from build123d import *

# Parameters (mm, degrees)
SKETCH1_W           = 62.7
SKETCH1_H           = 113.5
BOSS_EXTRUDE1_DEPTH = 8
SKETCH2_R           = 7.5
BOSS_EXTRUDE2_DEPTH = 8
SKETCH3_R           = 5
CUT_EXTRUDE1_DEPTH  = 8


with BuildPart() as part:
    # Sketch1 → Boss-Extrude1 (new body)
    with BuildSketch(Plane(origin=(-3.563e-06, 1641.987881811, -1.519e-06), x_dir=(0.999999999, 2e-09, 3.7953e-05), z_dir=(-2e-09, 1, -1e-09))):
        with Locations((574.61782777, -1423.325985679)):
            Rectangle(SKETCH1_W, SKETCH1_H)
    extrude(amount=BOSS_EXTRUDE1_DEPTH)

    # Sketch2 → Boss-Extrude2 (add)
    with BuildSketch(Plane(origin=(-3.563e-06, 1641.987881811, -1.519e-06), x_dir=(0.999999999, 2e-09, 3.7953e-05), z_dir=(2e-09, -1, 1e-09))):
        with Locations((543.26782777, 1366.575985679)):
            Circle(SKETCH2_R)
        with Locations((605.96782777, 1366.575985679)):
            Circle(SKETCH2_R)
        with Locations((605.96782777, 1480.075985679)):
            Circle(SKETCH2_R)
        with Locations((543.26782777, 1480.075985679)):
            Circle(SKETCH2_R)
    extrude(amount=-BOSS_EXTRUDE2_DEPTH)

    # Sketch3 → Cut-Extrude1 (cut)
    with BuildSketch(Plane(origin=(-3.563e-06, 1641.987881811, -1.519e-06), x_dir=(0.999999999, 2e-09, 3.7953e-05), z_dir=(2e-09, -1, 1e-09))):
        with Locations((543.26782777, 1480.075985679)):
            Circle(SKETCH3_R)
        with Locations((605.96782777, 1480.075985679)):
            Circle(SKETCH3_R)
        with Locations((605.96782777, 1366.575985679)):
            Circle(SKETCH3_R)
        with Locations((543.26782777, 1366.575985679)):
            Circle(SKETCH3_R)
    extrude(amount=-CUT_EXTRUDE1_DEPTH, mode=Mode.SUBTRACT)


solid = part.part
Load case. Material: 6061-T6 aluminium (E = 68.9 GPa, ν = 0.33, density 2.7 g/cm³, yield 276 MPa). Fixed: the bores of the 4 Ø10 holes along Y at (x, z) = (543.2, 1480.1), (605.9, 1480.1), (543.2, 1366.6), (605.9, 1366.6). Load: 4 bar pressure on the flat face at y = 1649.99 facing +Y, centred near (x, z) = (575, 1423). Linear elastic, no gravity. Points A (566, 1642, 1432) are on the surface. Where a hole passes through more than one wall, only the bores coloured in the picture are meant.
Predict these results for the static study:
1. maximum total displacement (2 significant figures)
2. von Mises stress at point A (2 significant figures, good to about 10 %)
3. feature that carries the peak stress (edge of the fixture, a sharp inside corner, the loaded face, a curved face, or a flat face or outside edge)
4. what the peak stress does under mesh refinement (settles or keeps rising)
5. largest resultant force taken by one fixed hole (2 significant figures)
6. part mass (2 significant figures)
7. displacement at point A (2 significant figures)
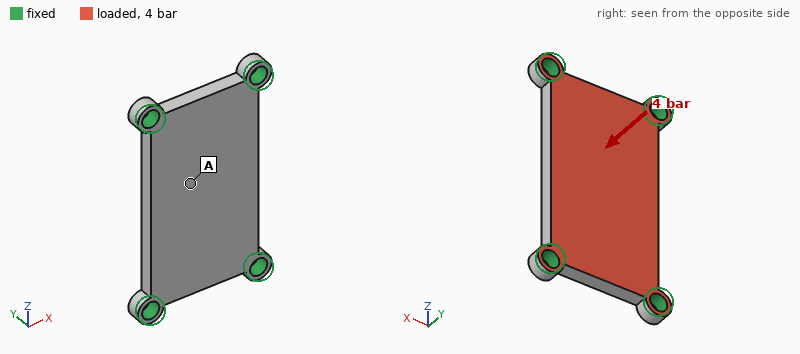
83 µm
20 MPa
edge of the fixture
keeps rising
730 N
160 g
77 µm
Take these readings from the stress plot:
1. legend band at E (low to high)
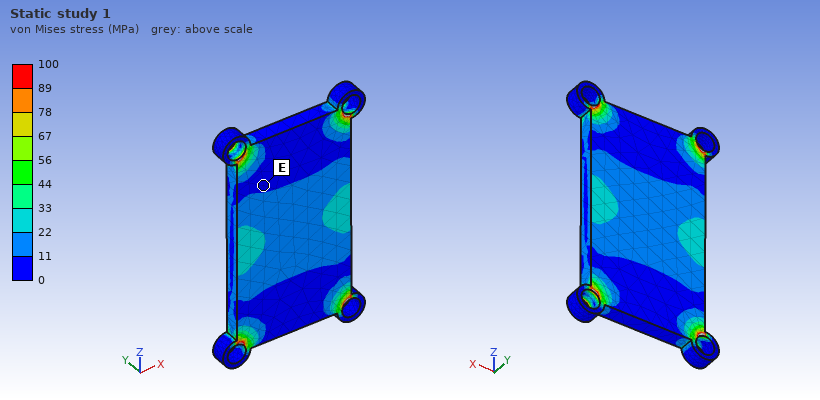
0 to 11 MPa
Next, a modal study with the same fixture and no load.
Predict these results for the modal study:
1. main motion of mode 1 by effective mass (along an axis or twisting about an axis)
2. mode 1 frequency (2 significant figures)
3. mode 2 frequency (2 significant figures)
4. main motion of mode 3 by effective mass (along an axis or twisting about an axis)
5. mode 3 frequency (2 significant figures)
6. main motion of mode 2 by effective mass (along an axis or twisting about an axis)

along Y
2700 Hz
4900 Hz
twisting about X
7300 Hz
twisting about Z
